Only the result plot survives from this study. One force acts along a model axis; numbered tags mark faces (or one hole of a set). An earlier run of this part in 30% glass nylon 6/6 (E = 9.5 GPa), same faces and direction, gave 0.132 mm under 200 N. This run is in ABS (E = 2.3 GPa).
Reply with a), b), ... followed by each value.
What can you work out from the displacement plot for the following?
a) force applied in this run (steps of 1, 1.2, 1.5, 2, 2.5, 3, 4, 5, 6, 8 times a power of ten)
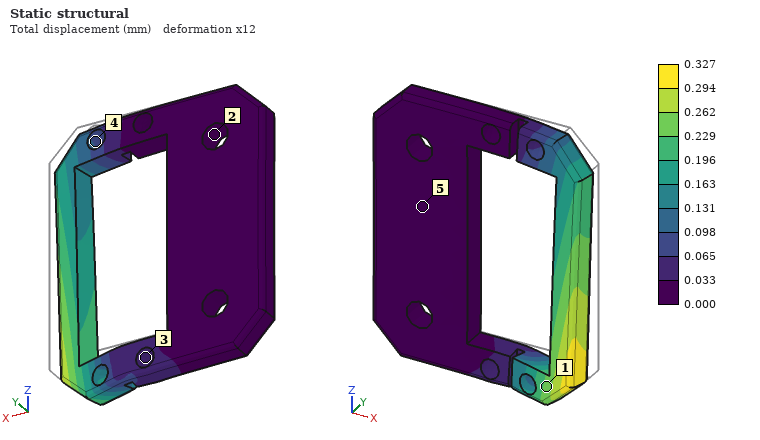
a) 120 N
